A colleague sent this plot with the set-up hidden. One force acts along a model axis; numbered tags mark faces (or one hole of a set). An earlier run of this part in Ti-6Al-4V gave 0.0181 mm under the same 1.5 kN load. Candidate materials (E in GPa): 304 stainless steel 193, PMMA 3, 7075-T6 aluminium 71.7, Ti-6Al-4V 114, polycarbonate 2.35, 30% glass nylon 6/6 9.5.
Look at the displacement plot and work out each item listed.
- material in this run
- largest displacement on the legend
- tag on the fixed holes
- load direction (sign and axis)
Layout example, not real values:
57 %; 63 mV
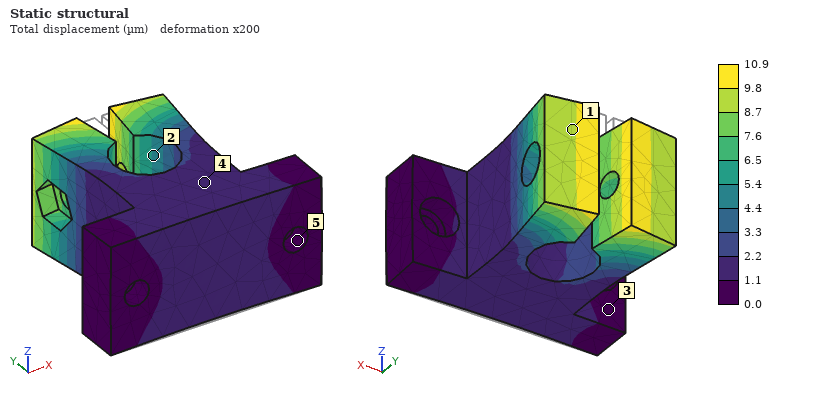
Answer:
304 stainless steel; 10.9 µm; 5; +Y
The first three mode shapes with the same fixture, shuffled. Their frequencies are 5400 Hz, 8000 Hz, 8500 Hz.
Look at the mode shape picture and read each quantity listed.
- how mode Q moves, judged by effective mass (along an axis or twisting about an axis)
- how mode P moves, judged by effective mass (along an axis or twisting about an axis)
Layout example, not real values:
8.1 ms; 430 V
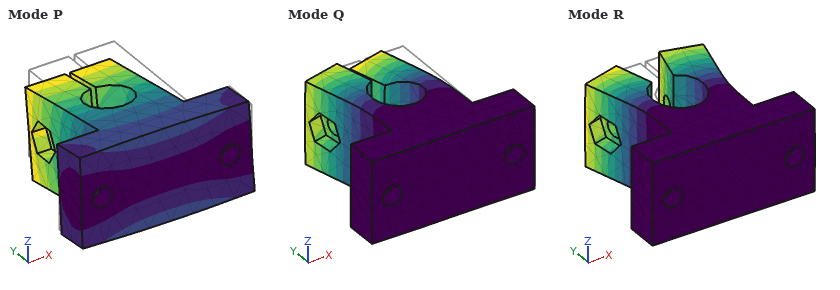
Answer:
along X; along Z
